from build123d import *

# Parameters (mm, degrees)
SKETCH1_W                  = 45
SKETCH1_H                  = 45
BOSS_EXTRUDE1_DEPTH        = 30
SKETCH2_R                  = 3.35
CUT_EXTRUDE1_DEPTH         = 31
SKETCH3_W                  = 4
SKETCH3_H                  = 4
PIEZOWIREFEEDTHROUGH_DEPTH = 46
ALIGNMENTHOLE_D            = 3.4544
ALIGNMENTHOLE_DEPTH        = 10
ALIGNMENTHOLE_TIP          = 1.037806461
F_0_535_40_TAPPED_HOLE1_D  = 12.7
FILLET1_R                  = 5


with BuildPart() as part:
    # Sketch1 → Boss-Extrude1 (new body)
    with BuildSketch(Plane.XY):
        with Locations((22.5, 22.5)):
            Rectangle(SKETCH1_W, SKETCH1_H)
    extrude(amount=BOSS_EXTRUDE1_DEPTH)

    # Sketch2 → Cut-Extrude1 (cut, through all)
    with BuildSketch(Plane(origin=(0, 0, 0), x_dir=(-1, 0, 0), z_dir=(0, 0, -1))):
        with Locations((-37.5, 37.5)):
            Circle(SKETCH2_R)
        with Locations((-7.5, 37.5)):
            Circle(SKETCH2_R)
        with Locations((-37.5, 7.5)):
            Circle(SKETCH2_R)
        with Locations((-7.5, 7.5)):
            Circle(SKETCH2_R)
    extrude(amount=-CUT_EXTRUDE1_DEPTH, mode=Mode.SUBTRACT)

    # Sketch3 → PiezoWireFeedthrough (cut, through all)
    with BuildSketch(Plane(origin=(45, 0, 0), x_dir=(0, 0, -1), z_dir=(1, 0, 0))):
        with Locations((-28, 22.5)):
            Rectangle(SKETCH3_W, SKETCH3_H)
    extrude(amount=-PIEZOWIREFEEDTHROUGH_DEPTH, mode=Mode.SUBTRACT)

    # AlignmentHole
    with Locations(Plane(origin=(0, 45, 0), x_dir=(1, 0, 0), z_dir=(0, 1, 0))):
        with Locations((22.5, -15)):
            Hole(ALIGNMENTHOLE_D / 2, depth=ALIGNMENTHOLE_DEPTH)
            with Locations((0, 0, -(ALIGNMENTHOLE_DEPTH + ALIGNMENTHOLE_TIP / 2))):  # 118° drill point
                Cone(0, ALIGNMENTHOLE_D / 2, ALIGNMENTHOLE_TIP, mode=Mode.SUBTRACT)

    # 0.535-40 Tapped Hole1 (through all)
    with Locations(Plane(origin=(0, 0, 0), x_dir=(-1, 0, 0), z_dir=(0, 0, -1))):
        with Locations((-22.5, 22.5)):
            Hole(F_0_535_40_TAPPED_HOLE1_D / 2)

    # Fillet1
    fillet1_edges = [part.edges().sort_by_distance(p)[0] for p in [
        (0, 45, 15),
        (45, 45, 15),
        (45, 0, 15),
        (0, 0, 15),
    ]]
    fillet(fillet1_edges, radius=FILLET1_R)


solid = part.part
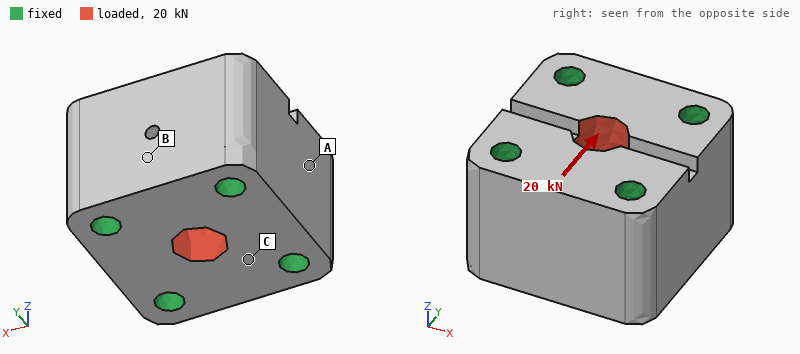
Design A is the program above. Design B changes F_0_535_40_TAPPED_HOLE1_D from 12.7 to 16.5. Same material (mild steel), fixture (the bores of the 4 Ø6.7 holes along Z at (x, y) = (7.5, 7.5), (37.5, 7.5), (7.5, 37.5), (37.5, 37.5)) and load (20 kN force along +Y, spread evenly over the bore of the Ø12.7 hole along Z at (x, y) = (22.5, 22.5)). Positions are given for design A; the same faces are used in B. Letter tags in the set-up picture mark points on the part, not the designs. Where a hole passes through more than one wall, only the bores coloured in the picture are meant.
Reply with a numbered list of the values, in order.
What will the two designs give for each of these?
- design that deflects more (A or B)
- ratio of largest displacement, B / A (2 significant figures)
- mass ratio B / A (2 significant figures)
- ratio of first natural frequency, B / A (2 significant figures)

1. A
2. 0.92
3. 0.95
4. 0.93
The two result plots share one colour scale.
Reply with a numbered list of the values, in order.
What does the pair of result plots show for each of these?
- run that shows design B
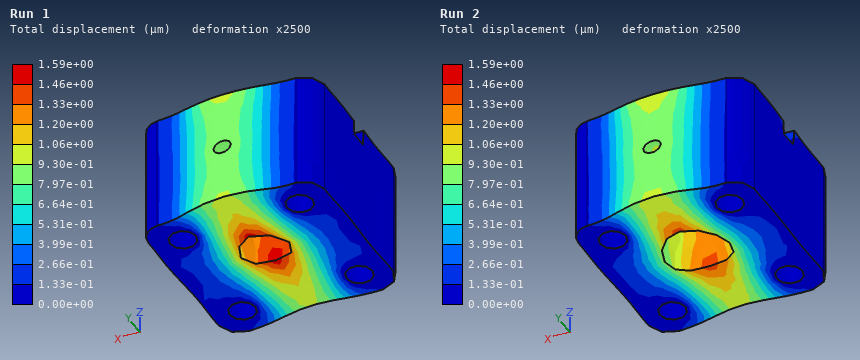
1. Run 2
